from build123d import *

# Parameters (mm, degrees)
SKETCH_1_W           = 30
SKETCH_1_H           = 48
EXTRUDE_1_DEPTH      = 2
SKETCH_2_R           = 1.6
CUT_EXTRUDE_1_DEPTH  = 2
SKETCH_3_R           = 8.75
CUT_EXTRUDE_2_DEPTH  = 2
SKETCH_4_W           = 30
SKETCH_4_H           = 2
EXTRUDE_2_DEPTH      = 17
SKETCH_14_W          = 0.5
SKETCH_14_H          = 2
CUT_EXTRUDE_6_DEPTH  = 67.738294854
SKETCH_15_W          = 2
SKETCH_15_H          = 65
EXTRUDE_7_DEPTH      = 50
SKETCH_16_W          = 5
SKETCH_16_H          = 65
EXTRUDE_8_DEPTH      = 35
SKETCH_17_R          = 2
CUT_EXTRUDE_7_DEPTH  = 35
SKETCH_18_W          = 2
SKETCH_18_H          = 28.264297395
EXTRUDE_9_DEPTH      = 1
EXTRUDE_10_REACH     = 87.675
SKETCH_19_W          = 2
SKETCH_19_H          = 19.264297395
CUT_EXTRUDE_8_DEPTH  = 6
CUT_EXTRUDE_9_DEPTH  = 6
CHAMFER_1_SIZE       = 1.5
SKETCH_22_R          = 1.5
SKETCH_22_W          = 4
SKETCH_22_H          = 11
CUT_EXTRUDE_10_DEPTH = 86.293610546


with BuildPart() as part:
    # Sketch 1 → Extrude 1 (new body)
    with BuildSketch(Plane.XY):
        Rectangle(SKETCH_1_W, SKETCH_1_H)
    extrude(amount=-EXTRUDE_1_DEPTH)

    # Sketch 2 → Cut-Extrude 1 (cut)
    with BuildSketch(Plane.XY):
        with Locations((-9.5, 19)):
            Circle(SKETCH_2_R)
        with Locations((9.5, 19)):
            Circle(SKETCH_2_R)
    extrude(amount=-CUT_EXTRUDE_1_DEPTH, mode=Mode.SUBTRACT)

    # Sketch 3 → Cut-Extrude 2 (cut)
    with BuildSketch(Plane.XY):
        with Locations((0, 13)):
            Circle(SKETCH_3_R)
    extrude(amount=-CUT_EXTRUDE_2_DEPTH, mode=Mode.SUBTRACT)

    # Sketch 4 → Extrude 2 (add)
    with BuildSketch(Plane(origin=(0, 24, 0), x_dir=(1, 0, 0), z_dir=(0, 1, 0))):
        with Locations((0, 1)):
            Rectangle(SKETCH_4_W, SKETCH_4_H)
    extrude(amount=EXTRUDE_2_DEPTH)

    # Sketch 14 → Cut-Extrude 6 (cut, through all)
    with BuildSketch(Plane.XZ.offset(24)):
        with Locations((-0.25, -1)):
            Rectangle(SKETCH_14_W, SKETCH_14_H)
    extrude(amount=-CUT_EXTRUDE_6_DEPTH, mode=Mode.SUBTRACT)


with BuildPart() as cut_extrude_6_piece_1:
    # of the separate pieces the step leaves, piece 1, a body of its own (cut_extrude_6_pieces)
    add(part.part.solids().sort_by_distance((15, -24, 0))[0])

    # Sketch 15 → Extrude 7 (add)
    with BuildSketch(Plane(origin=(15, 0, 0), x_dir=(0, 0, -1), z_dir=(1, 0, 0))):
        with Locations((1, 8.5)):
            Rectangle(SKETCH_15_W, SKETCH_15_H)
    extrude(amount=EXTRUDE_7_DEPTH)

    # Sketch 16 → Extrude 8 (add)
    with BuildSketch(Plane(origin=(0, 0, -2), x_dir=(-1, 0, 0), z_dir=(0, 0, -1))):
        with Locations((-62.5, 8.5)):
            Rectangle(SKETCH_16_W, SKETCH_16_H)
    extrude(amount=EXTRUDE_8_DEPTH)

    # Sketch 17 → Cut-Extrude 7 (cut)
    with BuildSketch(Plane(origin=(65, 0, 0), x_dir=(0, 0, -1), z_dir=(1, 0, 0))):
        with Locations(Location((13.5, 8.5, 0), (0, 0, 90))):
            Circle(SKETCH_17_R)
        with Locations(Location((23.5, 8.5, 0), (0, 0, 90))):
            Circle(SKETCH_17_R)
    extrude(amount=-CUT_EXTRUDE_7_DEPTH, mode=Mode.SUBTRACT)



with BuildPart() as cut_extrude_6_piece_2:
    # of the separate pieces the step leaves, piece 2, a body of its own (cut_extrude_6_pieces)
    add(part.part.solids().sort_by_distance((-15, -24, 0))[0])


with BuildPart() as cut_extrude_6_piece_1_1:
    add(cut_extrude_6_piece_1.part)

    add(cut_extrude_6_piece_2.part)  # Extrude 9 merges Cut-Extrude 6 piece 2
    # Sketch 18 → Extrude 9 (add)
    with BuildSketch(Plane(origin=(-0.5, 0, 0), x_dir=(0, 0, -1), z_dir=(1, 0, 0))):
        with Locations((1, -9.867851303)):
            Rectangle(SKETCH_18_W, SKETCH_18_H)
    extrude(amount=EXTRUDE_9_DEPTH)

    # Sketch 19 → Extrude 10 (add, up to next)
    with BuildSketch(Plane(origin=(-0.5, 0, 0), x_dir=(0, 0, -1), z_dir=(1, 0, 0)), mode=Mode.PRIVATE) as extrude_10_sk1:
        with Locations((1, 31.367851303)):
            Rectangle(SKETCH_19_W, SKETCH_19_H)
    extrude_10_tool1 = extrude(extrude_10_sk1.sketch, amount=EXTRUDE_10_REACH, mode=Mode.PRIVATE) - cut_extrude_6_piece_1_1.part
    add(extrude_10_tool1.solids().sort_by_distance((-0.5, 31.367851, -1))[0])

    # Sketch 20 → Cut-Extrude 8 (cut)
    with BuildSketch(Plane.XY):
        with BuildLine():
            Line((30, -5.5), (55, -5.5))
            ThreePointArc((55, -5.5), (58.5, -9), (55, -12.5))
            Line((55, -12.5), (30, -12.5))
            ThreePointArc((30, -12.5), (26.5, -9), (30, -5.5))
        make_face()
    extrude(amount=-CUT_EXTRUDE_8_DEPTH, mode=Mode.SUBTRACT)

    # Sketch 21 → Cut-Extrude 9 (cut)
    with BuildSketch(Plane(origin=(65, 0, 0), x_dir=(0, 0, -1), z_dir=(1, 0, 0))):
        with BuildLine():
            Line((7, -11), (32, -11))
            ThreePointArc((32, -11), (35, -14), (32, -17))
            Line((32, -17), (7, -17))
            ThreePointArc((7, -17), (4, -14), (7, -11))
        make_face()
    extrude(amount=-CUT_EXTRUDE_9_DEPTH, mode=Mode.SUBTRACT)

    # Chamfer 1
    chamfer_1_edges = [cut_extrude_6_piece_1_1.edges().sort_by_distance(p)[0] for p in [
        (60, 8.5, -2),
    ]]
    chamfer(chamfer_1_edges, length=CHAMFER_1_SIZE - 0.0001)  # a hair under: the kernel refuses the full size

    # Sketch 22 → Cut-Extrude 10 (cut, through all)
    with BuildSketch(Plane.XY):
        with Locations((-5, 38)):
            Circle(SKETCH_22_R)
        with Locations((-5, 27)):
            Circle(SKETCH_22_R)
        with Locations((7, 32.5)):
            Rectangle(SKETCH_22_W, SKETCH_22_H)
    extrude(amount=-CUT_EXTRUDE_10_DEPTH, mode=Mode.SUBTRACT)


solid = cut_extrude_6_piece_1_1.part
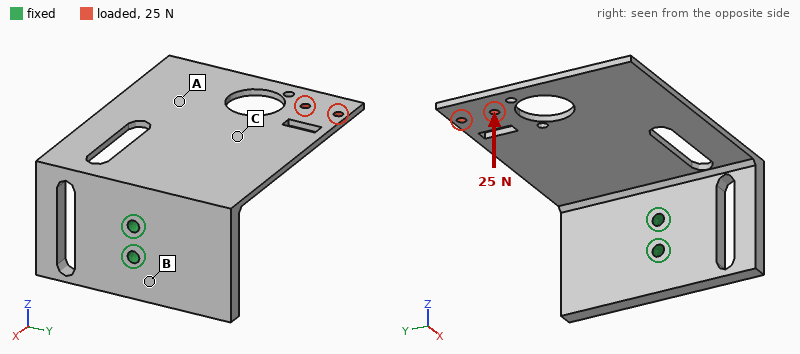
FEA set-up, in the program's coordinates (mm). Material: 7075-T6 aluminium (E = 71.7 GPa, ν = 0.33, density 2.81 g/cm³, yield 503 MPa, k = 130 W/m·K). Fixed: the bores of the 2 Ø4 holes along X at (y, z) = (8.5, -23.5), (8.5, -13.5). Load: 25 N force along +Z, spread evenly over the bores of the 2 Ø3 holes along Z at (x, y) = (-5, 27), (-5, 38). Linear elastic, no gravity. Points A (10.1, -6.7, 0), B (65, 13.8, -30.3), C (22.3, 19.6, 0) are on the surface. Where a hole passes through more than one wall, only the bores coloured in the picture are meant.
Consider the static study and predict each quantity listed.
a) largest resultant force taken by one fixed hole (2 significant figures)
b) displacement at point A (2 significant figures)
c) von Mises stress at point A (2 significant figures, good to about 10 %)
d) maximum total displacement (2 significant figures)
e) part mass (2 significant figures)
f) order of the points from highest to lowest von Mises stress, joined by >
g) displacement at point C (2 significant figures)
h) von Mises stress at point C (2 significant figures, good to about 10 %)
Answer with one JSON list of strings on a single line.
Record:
["91 N", "0.45 mm", "11 MPa", "1.2 mm", "56 g", "C > A > B", "0.36 mm", "19 MPa"]
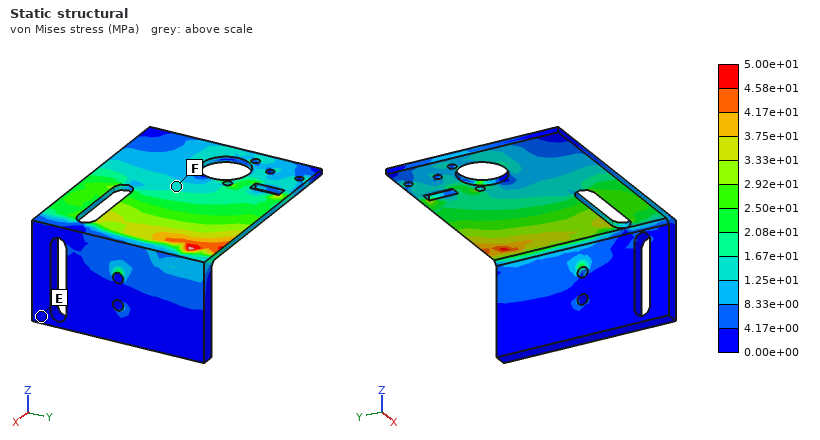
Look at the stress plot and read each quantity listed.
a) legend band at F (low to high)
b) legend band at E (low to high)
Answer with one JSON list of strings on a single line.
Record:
["1.25e+01 to 1.67e+01 MPa", "0.00e+00 to 4.17e+00 MPa"]
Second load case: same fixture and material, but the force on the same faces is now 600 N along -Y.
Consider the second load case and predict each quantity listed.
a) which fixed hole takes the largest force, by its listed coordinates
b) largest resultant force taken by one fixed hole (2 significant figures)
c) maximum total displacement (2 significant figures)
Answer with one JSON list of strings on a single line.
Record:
["(8.5, -13.5)", "1.1 kN", "1.1 mm"]
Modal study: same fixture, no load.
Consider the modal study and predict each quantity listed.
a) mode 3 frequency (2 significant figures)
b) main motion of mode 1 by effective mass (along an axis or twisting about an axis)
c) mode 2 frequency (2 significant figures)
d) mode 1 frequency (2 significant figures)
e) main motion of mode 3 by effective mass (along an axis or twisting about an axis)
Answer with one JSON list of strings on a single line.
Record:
["1100 Hz", "along Z", "760 Hz", "300 Hz", "along Y"]
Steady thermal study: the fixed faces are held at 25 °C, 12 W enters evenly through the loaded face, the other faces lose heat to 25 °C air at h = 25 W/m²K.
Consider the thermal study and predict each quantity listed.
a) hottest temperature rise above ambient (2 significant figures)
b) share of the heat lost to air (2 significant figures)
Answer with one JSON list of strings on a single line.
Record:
["79 K", "49 %"]
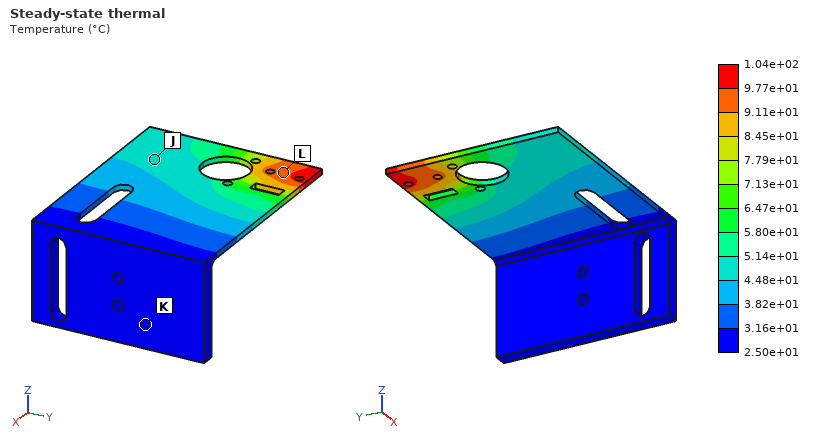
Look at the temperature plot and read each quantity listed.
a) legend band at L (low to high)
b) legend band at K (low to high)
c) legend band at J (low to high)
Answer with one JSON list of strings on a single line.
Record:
["9.11e+01 to 9.77e+01 °C", "2.50e+01 to 3.16e+01 °C", "4.48e+01 to 5.14e+01 °C"]
